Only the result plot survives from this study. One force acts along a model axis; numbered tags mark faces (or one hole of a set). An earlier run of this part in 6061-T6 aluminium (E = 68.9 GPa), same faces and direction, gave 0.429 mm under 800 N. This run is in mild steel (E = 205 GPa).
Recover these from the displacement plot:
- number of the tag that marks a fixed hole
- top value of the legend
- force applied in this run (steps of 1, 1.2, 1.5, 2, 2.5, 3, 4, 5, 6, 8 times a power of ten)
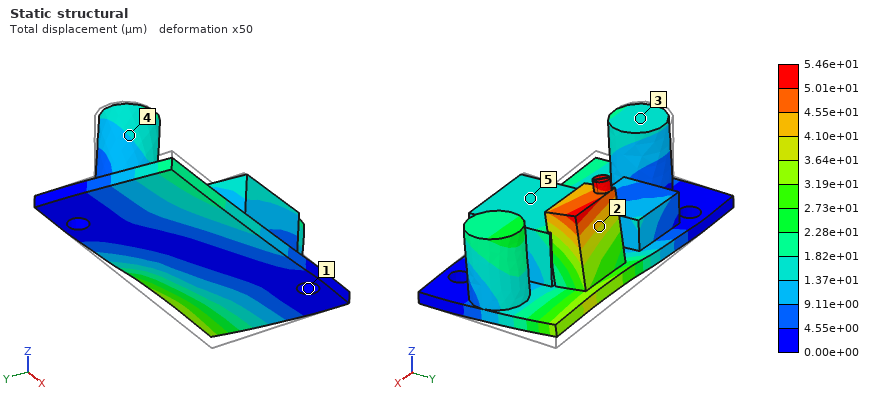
1
5.46e+01 µm
300 N
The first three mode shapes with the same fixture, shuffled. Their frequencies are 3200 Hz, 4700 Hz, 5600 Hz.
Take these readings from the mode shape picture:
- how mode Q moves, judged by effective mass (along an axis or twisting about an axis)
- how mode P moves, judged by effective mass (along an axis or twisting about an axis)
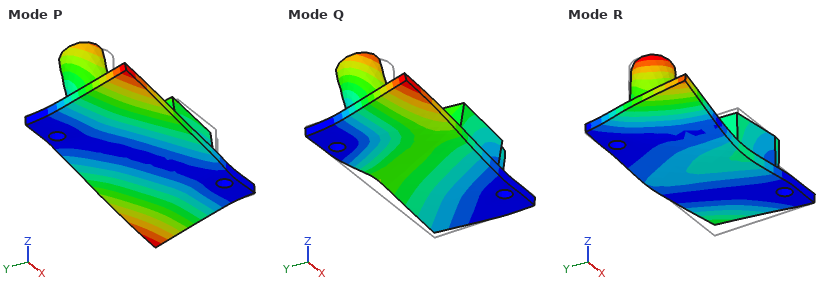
along Z
along Y
